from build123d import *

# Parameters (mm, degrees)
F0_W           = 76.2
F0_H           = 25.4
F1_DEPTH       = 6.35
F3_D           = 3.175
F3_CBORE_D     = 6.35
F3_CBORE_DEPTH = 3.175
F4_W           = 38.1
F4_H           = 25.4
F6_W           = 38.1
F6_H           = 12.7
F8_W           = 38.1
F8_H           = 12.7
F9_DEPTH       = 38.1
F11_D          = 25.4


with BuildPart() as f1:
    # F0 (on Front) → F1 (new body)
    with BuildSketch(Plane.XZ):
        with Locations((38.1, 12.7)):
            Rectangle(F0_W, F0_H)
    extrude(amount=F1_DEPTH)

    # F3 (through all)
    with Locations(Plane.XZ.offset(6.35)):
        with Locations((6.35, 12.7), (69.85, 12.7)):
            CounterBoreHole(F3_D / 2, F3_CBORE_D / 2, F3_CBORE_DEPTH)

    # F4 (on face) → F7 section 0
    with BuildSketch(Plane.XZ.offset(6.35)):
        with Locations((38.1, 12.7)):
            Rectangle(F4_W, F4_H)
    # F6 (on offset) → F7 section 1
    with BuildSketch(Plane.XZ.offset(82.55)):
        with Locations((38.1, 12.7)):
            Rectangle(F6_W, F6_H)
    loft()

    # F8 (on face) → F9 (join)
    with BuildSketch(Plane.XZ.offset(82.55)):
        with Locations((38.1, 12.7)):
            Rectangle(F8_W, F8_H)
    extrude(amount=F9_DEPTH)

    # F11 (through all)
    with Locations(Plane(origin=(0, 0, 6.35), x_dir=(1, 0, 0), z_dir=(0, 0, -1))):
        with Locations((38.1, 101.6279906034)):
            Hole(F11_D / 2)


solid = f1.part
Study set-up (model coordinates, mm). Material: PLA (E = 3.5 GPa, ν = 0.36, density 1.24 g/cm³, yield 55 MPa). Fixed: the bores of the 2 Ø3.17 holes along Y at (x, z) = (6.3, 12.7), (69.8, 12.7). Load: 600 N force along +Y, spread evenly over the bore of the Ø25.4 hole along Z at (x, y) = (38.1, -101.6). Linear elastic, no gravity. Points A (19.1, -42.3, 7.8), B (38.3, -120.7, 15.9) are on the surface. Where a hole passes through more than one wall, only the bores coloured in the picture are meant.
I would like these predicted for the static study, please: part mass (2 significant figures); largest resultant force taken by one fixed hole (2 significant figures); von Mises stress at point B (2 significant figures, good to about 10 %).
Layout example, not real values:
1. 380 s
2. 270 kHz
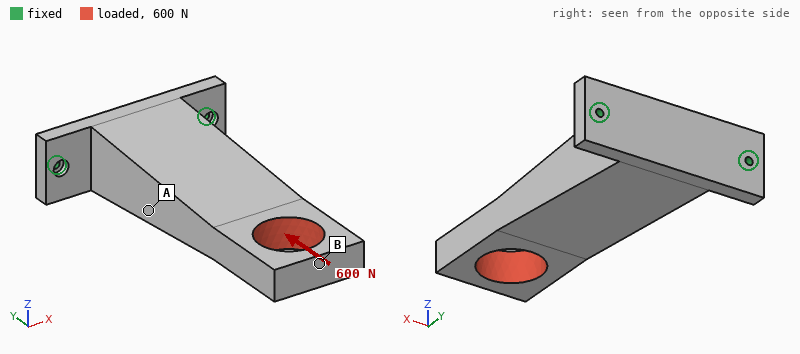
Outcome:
1. 98 g
2. 430 N
3. 3.8 MPa
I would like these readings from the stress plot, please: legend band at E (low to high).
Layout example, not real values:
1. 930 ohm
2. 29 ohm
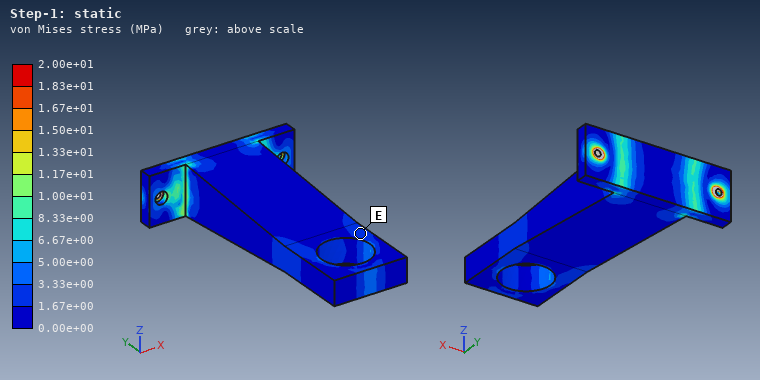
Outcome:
1. 1.67e+00 to 3.33e+00 MPa
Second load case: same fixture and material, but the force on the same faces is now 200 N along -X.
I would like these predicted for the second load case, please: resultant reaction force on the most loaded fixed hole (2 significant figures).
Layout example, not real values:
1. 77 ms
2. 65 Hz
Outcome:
1. 360 N
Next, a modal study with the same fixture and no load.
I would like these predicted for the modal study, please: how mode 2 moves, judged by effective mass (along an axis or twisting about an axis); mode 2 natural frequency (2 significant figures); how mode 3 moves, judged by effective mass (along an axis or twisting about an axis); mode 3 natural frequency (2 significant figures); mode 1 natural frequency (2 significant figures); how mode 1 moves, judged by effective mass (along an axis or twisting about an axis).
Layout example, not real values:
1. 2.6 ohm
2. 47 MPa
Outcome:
1. along X
2. 460 Hz
3. along Y
4. 1000 Hz
5. 110 Hz
6. along Z
